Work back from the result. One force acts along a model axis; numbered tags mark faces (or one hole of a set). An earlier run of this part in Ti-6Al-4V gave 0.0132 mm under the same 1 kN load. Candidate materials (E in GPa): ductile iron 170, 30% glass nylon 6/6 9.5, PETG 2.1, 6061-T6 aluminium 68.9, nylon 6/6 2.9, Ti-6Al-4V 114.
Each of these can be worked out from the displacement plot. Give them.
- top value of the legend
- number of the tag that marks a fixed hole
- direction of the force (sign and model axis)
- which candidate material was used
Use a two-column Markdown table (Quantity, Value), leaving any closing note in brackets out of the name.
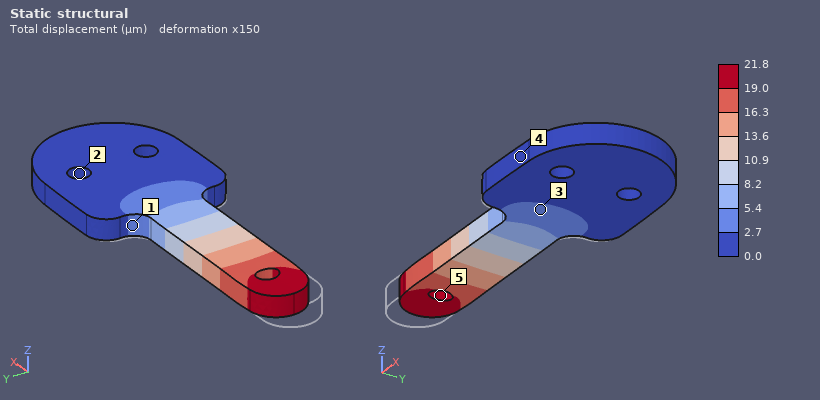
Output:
| Quantity | Value |
|---|---|
| top value of the legend | 21.8 µm |
| number of the tag that marks a fixed hole | 2 |
| direction of the force | +X |
| which candidate material was used | 6061-T6 aluminium |
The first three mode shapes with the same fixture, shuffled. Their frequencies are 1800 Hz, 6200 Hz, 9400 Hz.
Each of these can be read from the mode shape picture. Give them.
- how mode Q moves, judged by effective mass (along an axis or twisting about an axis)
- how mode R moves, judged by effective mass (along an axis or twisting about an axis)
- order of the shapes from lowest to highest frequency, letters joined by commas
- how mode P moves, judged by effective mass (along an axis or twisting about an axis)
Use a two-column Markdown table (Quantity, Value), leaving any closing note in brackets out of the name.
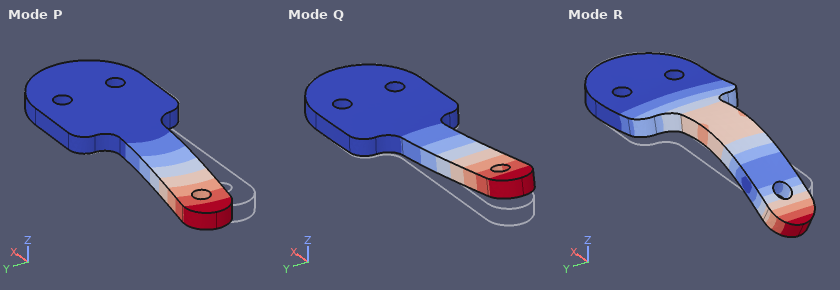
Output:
| Quantity | Value |
|---|---|
| how mode Q moves, judged by effective mass | along Z |
| how mode R moves, judged by effective mass | along Z |
| order of the shapes from lowest to highest frequency, letters joined by commas | Q, P, R |
| how mode P moves, judged by effective mass | along Y |
